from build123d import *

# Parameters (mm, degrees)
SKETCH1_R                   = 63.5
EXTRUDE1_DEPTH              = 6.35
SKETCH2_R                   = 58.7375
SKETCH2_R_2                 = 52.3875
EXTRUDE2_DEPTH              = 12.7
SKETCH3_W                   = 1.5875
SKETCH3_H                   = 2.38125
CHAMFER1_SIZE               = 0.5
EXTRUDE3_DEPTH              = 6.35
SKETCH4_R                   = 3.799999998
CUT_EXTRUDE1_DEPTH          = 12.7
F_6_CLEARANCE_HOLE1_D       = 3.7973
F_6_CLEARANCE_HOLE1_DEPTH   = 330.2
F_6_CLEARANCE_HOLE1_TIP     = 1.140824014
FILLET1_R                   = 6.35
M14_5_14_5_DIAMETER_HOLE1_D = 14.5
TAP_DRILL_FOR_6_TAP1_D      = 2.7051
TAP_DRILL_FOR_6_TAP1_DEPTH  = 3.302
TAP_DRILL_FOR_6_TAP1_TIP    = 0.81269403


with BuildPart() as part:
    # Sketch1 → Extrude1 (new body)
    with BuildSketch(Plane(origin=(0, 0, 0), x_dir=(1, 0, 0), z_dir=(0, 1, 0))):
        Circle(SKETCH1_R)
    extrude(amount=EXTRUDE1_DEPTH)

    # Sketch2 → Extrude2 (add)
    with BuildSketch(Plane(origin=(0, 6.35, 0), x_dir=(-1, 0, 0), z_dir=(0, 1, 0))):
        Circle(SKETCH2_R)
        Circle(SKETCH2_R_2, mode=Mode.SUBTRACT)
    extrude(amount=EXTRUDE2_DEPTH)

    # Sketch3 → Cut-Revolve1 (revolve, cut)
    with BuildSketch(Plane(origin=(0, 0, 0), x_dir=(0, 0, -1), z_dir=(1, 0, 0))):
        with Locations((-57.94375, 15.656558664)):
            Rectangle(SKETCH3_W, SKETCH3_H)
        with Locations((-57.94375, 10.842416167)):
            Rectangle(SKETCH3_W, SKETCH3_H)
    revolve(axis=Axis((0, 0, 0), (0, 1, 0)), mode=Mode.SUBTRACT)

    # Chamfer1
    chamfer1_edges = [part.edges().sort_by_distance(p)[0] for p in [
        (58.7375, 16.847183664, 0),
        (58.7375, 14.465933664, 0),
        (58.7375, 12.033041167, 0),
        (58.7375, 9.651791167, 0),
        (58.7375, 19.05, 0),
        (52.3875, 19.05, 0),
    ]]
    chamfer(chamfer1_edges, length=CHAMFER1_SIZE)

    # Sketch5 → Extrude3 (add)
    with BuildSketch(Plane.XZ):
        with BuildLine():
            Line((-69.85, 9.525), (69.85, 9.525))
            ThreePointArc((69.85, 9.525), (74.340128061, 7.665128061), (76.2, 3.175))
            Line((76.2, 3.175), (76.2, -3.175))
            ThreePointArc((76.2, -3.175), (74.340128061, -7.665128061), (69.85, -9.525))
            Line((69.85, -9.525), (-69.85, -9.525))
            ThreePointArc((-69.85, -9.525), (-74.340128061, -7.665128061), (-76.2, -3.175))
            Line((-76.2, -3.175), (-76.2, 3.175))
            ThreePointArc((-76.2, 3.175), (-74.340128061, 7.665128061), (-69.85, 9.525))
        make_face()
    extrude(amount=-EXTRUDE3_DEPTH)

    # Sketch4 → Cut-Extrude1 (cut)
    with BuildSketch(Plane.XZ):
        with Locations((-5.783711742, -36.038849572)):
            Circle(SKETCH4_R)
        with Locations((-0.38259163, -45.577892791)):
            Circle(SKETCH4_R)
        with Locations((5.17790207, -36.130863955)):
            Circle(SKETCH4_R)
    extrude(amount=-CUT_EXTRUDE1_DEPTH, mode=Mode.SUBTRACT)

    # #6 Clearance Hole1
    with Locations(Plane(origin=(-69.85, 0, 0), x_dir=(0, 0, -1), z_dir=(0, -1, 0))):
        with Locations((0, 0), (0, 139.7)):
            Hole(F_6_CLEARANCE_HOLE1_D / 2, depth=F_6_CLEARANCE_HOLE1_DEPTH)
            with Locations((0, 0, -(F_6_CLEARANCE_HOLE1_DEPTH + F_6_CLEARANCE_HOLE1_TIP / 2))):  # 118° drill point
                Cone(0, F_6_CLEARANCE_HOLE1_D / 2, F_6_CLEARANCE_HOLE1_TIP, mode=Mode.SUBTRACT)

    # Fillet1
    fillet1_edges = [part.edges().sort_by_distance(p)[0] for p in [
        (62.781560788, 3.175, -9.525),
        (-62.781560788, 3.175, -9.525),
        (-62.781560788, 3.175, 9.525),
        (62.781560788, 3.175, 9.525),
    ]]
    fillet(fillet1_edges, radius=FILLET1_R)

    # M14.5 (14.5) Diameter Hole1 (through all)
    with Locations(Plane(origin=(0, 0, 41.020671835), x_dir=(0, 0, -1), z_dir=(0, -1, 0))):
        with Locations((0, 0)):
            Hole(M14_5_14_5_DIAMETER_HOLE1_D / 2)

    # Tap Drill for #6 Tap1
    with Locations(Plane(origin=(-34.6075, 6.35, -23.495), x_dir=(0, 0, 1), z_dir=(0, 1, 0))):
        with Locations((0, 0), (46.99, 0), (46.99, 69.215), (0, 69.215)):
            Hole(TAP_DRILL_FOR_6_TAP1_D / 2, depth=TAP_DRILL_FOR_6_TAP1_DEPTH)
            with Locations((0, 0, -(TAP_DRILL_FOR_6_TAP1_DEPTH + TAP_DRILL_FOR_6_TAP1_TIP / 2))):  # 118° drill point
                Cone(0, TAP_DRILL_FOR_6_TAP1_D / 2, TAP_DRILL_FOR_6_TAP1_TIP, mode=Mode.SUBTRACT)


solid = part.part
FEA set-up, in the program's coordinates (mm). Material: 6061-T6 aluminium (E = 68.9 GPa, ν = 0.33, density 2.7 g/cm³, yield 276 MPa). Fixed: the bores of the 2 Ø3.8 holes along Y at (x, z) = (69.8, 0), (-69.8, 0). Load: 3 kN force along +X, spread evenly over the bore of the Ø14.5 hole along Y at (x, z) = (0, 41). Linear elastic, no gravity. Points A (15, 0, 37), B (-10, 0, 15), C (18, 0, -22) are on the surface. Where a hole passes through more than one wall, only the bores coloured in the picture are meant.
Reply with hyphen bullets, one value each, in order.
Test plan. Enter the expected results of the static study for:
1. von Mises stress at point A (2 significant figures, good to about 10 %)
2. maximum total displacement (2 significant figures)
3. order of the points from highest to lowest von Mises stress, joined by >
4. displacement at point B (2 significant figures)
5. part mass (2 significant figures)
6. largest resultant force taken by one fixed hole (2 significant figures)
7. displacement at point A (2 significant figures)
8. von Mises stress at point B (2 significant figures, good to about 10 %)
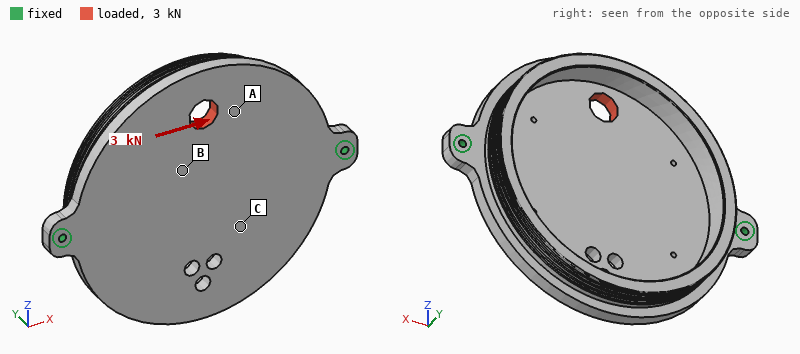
- 11 MPa
- 16 µm
- A > B > C
- 7.8 µm
- 290 g
- 1.7 kN
- 13 µm
- 6.1 MPa
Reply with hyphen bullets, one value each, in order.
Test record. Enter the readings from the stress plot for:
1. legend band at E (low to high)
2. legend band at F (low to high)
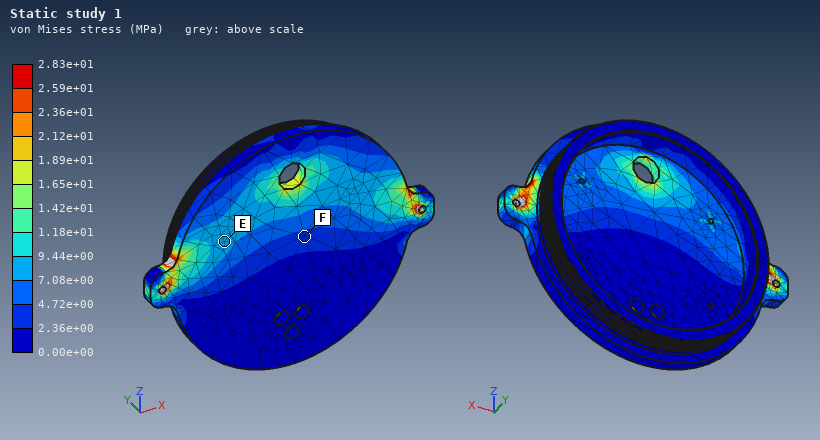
- 7.08e+00 to 9.44e+00 MPa
- 2.36e+00 to 4.72e+00 MPa
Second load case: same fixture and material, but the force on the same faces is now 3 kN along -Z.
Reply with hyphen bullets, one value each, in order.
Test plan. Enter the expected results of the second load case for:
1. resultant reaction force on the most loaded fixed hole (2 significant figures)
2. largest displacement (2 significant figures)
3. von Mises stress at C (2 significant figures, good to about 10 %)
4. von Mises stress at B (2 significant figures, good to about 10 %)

- 1.5 kN
- 19 µm
- 3.8 MPa
- 5.8 MPa
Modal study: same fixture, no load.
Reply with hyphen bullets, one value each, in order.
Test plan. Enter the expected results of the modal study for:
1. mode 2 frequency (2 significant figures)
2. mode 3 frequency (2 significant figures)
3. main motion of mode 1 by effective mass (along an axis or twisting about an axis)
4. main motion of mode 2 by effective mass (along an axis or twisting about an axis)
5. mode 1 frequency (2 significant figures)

- 1200 Hz
- 3100 Hz
- twisting about X
- along Y
- 670 Hz
